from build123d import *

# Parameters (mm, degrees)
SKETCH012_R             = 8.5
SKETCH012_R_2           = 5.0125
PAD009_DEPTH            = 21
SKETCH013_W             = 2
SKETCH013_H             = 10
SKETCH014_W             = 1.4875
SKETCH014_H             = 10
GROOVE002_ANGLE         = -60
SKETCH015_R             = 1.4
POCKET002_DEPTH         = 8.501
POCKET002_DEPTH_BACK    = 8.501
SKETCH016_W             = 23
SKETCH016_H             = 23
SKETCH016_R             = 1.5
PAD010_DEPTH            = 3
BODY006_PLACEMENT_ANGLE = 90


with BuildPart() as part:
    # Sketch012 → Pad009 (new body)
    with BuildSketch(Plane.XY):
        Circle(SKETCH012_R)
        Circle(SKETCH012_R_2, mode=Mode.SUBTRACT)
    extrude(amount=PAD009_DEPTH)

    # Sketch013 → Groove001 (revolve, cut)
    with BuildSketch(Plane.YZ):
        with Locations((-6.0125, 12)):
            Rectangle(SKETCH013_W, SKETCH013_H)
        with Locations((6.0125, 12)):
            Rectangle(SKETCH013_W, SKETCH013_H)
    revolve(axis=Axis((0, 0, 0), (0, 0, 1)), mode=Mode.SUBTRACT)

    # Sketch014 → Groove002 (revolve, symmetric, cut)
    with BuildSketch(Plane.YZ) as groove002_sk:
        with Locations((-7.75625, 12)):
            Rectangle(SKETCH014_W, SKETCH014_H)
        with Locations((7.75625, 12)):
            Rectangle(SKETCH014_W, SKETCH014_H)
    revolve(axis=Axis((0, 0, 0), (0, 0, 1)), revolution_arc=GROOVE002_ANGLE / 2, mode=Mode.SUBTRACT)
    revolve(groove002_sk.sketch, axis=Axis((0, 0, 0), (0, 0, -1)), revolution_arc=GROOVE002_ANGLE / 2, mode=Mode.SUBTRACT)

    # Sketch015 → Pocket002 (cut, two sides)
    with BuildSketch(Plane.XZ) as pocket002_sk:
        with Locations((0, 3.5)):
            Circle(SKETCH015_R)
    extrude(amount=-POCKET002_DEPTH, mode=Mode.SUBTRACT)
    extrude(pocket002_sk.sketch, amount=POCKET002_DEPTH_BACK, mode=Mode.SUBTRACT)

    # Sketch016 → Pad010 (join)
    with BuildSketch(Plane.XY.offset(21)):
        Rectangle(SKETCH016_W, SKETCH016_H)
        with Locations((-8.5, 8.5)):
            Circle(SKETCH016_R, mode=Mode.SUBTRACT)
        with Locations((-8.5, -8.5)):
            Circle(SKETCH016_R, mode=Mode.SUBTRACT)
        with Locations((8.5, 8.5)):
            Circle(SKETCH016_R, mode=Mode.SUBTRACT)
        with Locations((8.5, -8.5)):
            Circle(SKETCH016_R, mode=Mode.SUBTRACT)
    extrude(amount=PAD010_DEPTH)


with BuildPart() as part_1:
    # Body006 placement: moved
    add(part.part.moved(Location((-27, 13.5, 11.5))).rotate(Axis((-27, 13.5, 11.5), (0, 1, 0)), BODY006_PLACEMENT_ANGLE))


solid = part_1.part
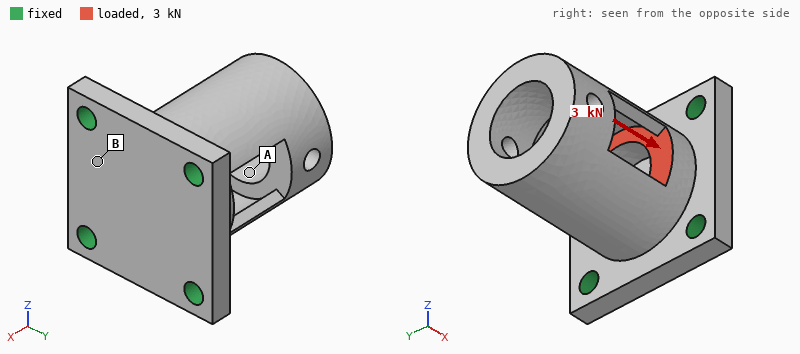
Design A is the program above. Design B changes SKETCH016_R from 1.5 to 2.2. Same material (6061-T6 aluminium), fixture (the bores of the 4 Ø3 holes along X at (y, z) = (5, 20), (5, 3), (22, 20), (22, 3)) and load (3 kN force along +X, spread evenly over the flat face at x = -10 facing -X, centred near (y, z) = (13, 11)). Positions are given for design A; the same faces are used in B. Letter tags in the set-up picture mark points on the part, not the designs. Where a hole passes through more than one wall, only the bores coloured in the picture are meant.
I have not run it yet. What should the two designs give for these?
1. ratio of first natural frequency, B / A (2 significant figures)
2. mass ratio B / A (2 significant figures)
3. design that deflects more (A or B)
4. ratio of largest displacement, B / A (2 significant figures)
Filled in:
1.0
0.97
A
0.72
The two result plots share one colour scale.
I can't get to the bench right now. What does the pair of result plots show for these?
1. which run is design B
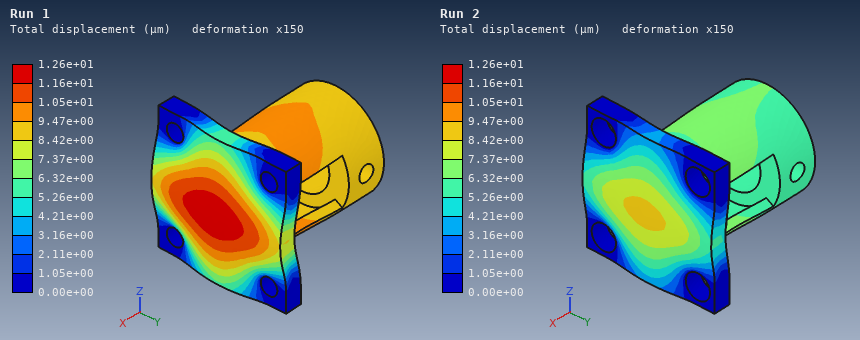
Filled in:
Run 2
